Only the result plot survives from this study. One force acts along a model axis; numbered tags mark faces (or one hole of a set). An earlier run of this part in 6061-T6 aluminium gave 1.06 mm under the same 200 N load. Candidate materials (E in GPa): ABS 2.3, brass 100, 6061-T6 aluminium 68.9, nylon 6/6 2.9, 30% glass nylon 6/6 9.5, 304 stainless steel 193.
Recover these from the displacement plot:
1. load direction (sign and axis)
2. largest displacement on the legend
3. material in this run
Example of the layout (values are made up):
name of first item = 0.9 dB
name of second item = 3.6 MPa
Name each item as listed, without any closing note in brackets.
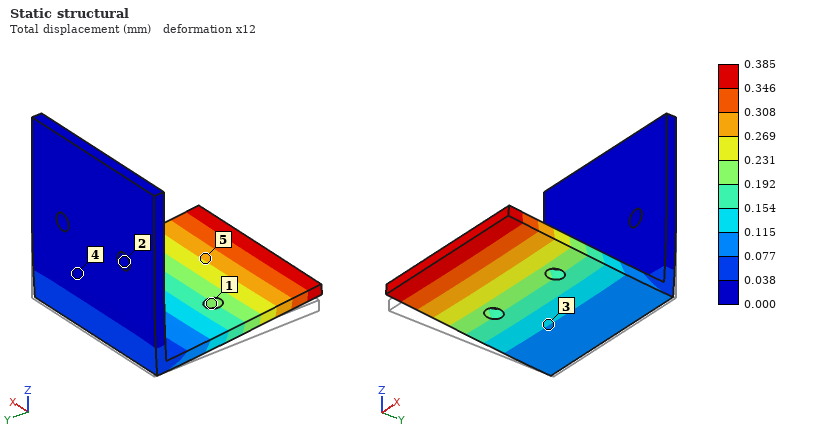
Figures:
load direction = +Z
largest displacement on the legend = 0.385 mm
material in this run = 304 stainless steel
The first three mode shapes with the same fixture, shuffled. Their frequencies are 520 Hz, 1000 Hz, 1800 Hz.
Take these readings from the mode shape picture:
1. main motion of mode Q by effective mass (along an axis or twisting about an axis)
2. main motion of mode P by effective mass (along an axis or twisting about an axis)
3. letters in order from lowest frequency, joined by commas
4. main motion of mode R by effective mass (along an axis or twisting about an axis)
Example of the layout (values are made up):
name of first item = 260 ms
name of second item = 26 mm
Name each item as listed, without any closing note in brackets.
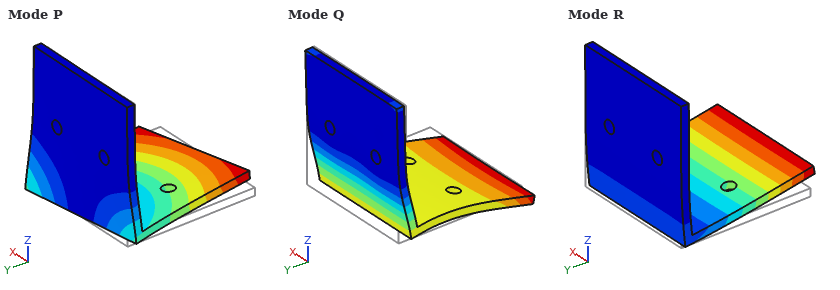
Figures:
main motion of mode Q by effective mass = along Y
main motion of mode P by effective mass = along X
letters in order from lowest frequency, joined by commas = R, P, Q
main motion of mode R by effective mass = along Z
